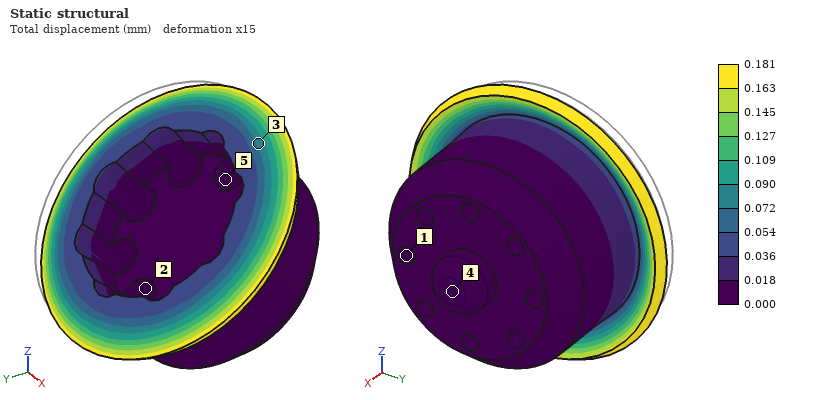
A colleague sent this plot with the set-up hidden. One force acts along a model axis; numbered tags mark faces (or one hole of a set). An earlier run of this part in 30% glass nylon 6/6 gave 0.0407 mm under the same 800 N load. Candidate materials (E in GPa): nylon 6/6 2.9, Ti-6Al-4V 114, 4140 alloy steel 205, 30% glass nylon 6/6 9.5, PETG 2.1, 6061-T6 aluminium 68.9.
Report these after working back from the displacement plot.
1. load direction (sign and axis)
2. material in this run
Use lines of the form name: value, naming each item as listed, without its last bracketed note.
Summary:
load direction: +X
material in this run: PETG
